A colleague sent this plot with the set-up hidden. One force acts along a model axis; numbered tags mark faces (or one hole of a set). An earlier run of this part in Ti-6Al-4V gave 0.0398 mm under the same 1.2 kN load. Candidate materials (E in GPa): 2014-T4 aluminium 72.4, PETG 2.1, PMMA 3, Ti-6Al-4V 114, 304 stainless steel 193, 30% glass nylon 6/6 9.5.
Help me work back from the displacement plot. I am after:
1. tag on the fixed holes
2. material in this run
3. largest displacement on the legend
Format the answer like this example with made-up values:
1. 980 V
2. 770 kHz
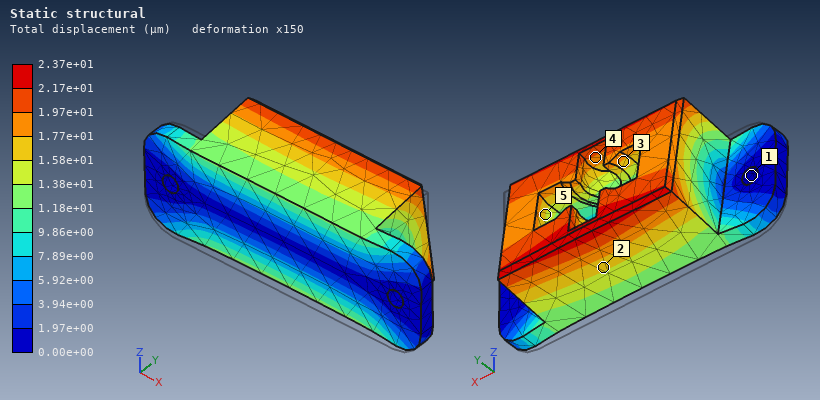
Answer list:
1. 1
2. 304 stainless steel
3. 2.37e+01 µm
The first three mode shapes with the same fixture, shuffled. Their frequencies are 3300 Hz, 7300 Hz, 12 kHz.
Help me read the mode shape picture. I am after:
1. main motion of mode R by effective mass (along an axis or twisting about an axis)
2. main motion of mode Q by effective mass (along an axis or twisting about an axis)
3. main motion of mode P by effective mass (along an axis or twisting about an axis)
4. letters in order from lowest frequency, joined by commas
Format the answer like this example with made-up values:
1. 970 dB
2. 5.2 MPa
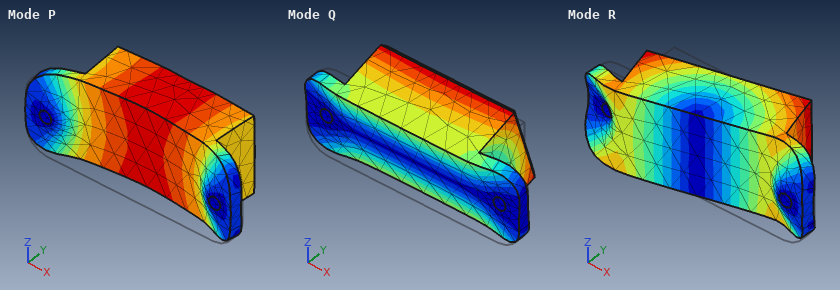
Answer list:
1. along X
2. along Z
3. along Y
4. Q, P, R
